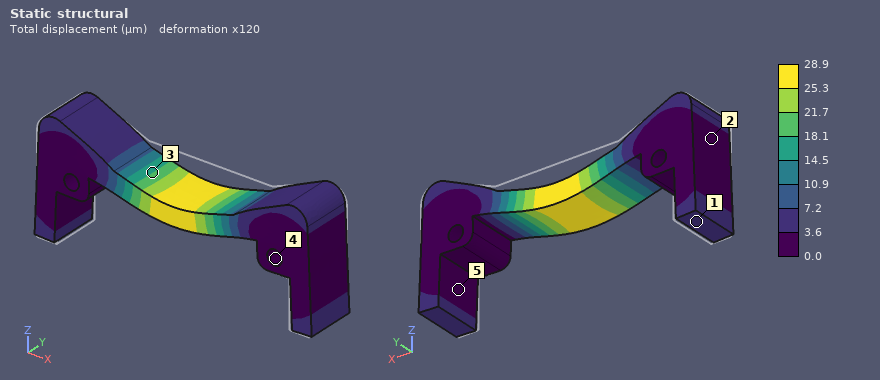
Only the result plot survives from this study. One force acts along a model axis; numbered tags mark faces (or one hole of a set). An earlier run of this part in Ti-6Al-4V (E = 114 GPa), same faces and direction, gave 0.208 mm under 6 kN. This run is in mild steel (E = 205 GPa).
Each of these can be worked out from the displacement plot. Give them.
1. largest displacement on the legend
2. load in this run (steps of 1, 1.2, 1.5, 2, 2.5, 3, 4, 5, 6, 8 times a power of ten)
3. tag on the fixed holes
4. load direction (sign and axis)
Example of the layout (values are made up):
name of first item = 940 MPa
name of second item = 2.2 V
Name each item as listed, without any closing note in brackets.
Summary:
largest displacement on the legend = 28.9 µm
load in this run = 1.5 kN
tag on the fixed holes = 4
load direction = -Z
